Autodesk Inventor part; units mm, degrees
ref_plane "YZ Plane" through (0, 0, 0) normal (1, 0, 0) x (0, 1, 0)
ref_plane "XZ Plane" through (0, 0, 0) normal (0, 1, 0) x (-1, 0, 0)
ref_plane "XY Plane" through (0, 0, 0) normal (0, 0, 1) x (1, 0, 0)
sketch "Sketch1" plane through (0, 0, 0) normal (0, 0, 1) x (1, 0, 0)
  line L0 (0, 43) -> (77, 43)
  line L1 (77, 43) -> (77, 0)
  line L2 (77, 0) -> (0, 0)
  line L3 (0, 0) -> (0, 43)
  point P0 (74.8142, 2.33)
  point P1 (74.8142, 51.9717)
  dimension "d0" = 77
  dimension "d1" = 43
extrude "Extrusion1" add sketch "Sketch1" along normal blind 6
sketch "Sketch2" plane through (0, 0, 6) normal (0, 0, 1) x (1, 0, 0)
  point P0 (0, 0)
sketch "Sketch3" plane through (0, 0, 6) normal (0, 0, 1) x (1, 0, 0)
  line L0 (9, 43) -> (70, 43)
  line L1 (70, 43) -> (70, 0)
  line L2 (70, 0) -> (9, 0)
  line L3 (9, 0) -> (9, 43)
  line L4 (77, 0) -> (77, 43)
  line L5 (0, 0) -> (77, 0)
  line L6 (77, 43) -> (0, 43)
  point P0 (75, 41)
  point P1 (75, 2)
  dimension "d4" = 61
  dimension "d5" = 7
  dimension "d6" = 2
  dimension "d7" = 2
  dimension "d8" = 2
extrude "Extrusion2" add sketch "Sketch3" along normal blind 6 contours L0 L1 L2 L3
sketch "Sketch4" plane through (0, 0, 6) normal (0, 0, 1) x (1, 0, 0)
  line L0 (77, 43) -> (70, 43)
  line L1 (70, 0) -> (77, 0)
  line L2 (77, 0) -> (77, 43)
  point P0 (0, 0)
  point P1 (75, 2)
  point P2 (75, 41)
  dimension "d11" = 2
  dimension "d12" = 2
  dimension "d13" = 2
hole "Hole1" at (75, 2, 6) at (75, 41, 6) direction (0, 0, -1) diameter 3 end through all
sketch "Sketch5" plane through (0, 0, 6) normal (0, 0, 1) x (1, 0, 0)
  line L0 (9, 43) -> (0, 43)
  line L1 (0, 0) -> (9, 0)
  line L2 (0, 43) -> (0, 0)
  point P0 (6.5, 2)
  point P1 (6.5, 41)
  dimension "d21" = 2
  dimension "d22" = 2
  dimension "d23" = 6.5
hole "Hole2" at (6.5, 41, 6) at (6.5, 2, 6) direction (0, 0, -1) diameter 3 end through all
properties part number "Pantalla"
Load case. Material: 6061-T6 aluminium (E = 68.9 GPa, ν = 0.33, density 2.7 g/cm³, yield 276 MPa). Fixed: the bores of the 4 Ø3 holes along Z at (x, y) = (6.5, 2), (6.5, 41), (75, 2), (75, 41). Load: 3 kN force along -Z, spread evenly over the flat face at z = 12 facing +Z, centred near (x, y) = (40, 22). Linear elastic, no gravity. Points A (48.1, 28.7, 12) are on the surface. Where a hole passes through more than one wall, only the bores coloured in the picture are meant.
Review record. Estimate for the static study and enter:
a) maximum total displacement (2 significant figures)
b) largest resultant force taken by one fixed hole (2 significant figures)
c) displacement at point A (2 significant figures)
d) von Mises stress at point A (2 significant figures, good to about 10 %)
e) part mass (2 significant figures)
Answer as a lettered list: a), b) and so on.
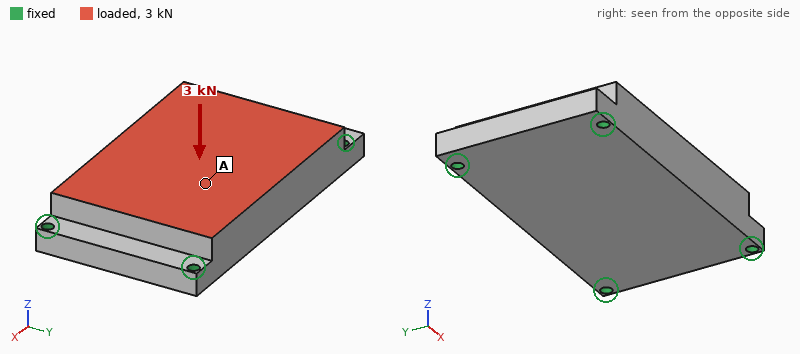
a) 24 µm
b) 1.0 kN
c) 21 µm
d) 16 MPa
e) 96 g
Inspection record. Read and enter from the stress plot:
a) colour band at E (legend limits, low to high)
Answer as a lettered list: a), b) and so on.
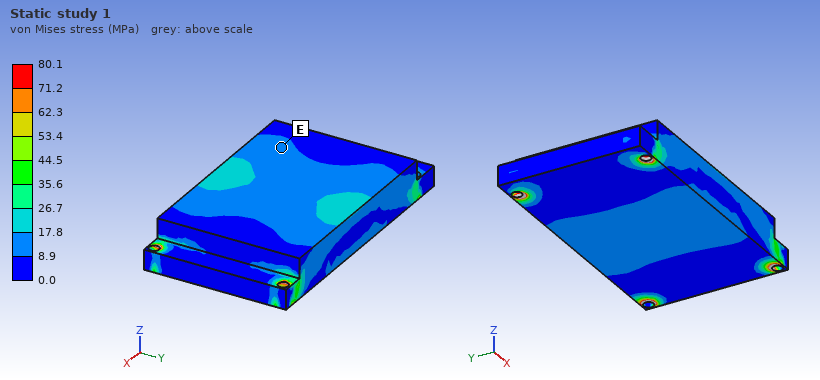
a) 8.9 to 17.8 MPa
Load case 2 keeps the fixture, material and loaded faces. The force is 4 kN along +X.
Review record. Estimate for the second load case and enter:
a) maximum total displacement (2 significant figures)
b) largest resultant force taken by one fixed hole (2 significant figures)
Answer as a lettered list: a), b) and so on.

a) 5.3 µm
b) 1.1 kN
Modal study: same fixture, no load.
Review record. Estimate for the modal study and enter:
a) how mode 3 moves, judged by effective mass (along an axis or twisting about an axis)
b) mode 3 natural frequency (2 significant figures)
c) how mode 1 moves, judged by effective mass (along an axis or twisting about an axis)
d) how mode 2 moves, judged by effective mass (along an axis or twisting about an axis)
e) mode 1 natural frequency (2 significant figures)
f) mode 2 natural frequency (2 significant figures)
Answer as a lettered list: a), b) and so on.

a) along Y
b) 14 kHz
c) along Z
d) twisting about X
e) 6900 Hz
f) 11 kHz
